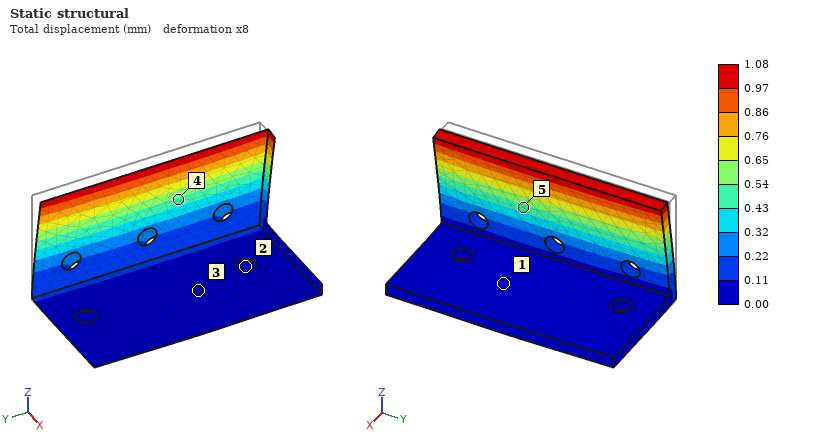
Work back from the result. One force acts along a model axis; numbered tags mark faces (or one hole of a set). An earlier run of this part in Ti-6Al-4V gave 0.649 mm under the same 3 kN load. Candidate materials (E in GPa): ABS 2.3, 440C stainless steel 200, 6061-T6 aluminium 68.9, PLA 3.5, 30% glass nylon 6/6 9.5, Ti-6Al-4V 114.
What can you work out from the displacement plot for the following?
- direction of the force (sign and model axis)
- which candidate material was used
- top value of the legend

+X
6061-T6 aluminium
1.08 mm
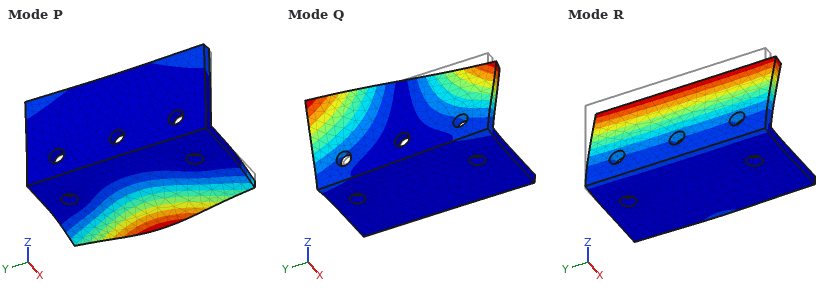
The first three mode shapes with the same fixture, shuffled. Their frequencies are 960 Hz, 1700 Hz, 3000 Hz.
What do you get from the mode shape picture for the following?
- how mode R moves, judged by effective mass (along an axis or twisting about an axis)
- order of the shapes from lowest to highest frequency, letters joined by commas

along X
R, Q, P
